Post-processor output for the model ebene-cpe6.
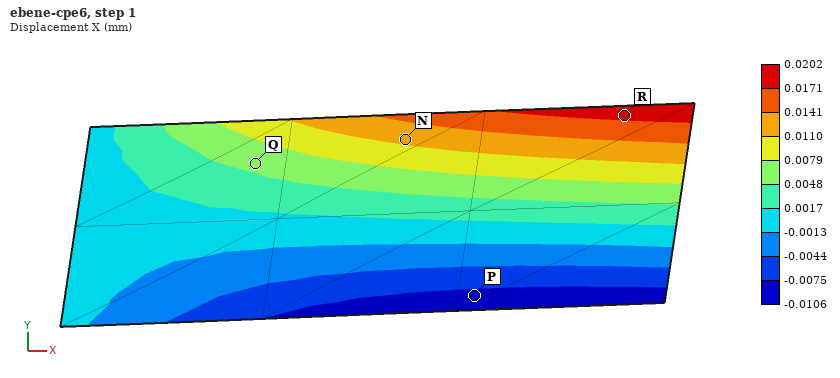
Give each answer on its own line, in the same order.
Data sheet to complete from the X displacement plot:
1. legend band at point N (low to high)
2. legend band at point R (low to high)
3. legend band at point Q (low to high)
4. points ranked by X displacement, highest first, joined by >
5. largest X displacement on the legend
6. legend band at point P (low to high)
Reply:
0.0110 to 0.0141 mm
0.0171 to 0.0202 mm
0.0048 to 0.0079 mm
R > N > Q > P
0.0202 mm
-0.0106 to -0.0075 mm
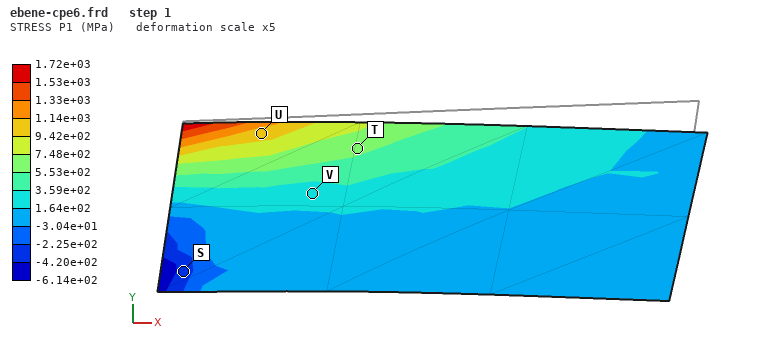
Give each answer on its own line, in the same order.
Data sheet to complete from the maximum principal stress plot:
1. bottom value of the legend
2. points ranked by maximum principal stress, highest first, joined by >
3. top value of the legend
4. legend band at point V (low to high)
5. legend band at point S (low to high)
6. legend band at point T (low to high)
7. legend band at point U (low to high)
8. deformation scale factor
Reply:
-6.14e+02 MPa
U > T > V > S
1.72e+03 MPa
1.64e+02 to 3.59e+02 MPa
-4.20e+02 to -2.25e+02 MPa
5.53e+02 to 7.48e+02 MPa
9.42e+02 to 1.14e+03 MPa
5
